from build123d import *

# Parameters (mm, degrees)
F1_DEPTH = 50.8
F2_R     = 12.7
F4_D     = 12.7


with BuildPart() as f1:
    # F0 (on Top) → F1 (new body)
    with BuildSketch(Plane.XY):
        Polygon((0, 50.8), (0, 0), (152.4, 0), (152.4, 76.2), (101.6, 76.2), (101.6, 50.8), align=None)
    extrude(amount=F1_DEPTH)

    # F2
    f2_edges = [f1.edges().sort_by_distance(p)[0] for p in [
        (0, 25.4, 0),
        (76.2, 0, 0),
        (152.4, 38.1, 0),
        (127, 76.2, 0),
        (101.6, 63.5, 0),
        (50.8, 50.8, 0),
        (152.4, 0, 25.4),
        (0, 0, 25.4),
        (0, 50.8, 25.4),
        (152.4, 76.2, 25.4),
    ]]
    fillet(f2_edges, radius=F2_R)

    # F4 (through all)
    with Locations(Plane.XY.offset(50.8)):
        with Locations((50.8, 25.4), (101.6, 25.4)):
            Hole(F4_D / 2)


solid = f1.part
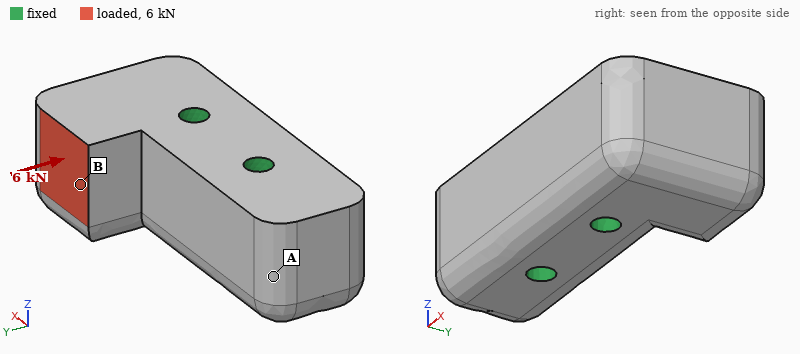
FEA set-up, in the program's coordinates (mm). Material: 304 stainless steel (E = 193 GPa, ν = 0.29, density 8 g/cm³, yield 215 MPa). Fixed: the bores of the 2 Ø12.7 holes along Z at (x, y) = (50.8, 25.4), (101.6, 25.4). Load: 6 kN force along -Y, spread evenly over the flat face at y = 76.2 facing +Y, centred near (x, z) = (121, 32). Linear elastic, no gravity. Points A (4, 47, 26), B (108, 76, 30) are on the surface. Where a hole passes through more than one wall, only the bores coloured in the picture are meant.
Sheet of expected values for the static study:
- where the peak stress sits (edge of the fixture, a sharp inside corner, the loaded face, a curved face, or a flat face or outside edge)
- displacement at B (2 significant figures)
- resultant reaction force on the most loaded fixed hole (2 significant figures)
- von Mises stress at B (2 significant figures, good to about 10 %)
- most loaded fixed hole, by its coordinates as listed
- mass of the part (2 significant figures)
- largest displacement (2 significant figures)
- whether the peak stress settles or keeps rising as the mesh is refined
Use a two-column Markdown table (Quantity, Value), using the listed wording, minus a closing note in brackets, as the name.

| Quantity | Value |
|---|---|
| where the peak stress sits | edge of the fixture |
| displacement at B | 2.3 µm |
| resultant reaction force on the most loaded fixed hole | 7.2 kN |
| von Mises stress at B | 3.7 MPa |
| most loaded fixed hole, by its coordinates as listed | (101.6, 25.4) |
| mass of the part | 3.4 kg |
| largest displacement | 3.3 µm |
| whether the peak stress settles or keeps rising as the mesh is refined | keeps rising |
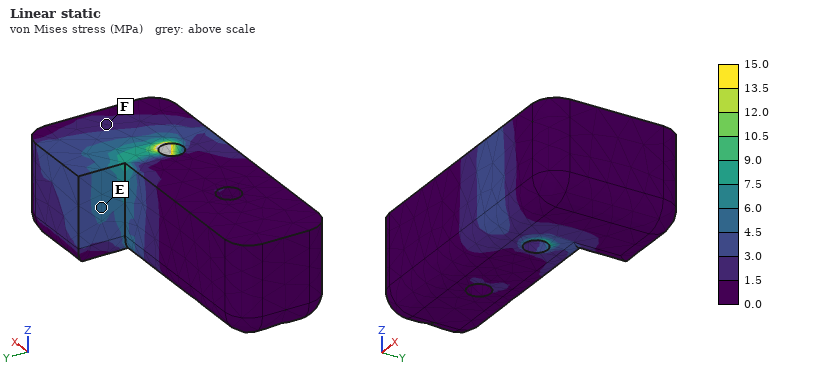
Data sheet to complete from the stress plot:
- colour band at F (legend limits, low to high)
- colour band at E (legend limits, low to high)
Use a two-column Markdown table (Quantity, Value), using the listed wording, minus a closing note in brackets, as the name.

| Quantity | Value |
|---|---|
| colour band at F | 1.5 to 3.0 MPa |
| colour band at E | 4.5 to 6.0 MPa |
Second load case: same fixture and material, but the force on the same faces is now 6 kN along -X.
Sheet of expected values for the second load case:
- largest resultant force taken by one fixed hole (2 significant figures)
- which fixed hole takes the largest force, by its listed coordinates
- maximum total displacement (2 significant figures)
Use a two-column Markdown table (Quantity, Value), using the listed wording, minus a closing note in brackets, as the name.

| Quantity | Value |
|---|---|
| largest resultant force taken by one fixed hole | 5.8 kN |
| which fixed hole takes the largest force, by its listed coordinates | (101.6, 25.4) |
| maximum total displacement | 9.2 µm |
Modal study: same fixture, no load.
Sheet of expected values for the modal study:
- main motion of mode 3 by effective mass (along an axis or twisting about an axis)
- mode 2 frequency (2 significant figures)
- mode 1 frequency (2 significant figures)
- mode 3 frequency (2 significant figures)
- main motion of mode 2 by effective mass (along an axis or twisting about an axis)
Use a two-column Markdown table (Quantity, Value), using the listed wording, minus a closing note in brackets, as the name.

| Quantity | Value |
|---|---|
| main motion of mode 3 by effective mass | along Y |
| mode 2 frequency | 7300 Hz |
| mode 1 frequency | 5700 Hz |
| mode 3 frequency | 8200 Hz |
| main motion of mode 2 by effective mass | along Z |
